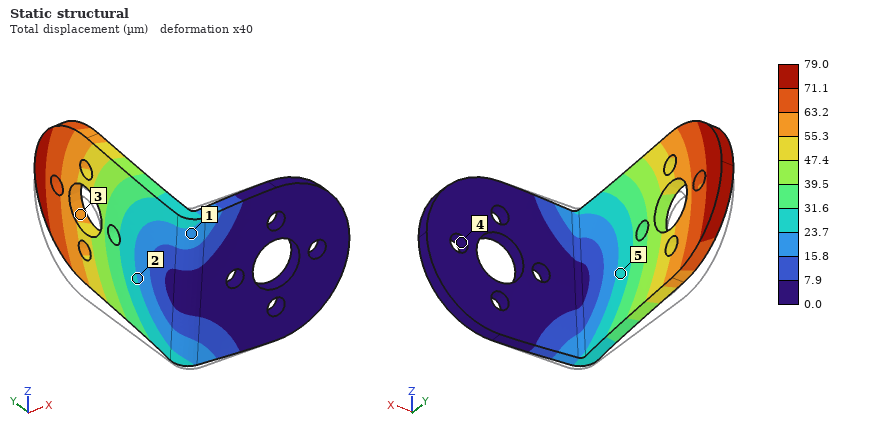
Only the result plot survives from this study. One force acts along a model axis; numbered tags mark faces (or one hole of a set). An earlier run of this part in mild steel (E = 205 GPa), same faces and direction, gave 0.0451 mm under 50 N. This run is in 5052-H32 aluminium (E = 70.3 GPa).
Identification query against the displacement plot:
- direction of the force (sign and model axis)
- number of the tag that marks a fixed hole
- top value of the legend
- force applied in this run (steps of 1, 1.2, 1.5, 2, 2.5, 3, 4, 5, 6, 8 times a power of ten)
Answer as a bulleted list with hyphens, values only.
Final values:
- +Z
- 4
- 79.0 µm
- 30 N
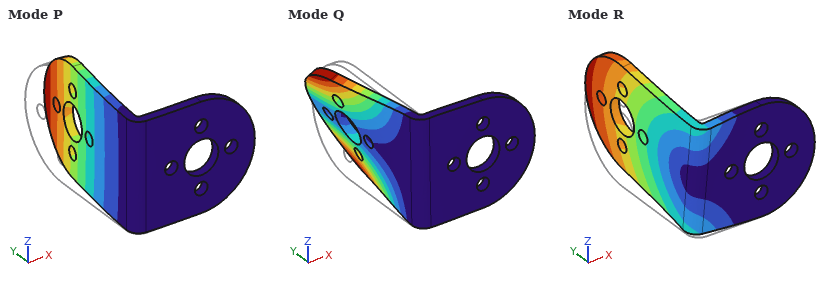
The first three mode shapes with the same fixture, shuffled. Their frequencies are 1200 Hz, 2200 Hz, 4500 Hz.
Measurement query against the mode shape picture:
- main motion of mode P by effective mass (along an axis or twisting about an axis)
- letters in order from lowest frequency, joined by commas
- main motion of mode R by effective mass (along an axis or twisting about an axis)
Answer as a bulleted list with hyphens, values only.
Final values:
- along X
- P, R, Q
- along Z
